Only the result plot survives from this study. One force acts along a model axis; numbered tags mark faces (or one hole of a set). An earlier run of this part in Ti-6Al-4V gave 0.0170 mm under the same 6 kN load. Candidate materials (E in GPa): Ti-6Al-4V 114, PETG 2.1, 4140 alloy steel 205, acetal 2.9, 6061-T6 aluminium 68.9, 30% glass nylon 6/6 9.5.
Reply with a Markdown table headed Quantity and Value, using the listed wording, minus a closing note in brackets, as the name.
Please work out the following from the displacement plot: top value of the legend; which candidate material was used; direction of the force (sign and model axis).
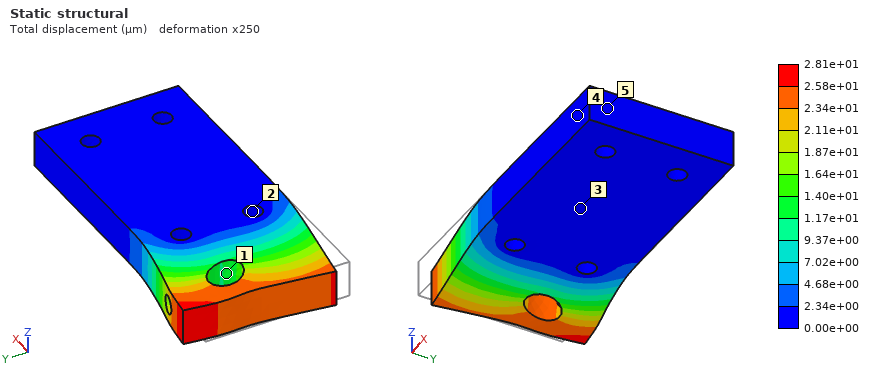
| Quantity | Value |
|---|---|
| top value of the legend | 2.81e+01 µm |
| which candidate material was used | 6061-T6 aluminium |
| direction of the force | +Y |
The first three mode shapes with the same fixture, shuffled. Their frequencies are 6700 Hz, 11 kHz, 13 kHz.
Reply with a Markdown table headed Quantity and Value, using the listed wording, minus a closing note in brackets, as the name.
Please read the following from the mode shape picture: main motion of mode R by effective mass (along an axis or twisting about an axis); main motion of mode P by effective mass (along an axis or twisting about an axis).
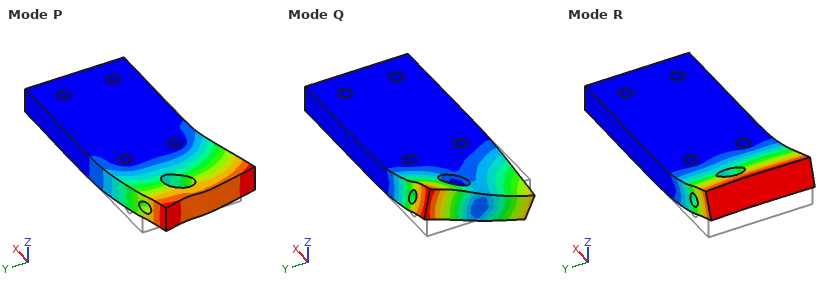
| Quantity | Value |
|---|---|
| main motion of mode R by effective mass | along Z |
| main motion of mode P by effective mass | along Y |
